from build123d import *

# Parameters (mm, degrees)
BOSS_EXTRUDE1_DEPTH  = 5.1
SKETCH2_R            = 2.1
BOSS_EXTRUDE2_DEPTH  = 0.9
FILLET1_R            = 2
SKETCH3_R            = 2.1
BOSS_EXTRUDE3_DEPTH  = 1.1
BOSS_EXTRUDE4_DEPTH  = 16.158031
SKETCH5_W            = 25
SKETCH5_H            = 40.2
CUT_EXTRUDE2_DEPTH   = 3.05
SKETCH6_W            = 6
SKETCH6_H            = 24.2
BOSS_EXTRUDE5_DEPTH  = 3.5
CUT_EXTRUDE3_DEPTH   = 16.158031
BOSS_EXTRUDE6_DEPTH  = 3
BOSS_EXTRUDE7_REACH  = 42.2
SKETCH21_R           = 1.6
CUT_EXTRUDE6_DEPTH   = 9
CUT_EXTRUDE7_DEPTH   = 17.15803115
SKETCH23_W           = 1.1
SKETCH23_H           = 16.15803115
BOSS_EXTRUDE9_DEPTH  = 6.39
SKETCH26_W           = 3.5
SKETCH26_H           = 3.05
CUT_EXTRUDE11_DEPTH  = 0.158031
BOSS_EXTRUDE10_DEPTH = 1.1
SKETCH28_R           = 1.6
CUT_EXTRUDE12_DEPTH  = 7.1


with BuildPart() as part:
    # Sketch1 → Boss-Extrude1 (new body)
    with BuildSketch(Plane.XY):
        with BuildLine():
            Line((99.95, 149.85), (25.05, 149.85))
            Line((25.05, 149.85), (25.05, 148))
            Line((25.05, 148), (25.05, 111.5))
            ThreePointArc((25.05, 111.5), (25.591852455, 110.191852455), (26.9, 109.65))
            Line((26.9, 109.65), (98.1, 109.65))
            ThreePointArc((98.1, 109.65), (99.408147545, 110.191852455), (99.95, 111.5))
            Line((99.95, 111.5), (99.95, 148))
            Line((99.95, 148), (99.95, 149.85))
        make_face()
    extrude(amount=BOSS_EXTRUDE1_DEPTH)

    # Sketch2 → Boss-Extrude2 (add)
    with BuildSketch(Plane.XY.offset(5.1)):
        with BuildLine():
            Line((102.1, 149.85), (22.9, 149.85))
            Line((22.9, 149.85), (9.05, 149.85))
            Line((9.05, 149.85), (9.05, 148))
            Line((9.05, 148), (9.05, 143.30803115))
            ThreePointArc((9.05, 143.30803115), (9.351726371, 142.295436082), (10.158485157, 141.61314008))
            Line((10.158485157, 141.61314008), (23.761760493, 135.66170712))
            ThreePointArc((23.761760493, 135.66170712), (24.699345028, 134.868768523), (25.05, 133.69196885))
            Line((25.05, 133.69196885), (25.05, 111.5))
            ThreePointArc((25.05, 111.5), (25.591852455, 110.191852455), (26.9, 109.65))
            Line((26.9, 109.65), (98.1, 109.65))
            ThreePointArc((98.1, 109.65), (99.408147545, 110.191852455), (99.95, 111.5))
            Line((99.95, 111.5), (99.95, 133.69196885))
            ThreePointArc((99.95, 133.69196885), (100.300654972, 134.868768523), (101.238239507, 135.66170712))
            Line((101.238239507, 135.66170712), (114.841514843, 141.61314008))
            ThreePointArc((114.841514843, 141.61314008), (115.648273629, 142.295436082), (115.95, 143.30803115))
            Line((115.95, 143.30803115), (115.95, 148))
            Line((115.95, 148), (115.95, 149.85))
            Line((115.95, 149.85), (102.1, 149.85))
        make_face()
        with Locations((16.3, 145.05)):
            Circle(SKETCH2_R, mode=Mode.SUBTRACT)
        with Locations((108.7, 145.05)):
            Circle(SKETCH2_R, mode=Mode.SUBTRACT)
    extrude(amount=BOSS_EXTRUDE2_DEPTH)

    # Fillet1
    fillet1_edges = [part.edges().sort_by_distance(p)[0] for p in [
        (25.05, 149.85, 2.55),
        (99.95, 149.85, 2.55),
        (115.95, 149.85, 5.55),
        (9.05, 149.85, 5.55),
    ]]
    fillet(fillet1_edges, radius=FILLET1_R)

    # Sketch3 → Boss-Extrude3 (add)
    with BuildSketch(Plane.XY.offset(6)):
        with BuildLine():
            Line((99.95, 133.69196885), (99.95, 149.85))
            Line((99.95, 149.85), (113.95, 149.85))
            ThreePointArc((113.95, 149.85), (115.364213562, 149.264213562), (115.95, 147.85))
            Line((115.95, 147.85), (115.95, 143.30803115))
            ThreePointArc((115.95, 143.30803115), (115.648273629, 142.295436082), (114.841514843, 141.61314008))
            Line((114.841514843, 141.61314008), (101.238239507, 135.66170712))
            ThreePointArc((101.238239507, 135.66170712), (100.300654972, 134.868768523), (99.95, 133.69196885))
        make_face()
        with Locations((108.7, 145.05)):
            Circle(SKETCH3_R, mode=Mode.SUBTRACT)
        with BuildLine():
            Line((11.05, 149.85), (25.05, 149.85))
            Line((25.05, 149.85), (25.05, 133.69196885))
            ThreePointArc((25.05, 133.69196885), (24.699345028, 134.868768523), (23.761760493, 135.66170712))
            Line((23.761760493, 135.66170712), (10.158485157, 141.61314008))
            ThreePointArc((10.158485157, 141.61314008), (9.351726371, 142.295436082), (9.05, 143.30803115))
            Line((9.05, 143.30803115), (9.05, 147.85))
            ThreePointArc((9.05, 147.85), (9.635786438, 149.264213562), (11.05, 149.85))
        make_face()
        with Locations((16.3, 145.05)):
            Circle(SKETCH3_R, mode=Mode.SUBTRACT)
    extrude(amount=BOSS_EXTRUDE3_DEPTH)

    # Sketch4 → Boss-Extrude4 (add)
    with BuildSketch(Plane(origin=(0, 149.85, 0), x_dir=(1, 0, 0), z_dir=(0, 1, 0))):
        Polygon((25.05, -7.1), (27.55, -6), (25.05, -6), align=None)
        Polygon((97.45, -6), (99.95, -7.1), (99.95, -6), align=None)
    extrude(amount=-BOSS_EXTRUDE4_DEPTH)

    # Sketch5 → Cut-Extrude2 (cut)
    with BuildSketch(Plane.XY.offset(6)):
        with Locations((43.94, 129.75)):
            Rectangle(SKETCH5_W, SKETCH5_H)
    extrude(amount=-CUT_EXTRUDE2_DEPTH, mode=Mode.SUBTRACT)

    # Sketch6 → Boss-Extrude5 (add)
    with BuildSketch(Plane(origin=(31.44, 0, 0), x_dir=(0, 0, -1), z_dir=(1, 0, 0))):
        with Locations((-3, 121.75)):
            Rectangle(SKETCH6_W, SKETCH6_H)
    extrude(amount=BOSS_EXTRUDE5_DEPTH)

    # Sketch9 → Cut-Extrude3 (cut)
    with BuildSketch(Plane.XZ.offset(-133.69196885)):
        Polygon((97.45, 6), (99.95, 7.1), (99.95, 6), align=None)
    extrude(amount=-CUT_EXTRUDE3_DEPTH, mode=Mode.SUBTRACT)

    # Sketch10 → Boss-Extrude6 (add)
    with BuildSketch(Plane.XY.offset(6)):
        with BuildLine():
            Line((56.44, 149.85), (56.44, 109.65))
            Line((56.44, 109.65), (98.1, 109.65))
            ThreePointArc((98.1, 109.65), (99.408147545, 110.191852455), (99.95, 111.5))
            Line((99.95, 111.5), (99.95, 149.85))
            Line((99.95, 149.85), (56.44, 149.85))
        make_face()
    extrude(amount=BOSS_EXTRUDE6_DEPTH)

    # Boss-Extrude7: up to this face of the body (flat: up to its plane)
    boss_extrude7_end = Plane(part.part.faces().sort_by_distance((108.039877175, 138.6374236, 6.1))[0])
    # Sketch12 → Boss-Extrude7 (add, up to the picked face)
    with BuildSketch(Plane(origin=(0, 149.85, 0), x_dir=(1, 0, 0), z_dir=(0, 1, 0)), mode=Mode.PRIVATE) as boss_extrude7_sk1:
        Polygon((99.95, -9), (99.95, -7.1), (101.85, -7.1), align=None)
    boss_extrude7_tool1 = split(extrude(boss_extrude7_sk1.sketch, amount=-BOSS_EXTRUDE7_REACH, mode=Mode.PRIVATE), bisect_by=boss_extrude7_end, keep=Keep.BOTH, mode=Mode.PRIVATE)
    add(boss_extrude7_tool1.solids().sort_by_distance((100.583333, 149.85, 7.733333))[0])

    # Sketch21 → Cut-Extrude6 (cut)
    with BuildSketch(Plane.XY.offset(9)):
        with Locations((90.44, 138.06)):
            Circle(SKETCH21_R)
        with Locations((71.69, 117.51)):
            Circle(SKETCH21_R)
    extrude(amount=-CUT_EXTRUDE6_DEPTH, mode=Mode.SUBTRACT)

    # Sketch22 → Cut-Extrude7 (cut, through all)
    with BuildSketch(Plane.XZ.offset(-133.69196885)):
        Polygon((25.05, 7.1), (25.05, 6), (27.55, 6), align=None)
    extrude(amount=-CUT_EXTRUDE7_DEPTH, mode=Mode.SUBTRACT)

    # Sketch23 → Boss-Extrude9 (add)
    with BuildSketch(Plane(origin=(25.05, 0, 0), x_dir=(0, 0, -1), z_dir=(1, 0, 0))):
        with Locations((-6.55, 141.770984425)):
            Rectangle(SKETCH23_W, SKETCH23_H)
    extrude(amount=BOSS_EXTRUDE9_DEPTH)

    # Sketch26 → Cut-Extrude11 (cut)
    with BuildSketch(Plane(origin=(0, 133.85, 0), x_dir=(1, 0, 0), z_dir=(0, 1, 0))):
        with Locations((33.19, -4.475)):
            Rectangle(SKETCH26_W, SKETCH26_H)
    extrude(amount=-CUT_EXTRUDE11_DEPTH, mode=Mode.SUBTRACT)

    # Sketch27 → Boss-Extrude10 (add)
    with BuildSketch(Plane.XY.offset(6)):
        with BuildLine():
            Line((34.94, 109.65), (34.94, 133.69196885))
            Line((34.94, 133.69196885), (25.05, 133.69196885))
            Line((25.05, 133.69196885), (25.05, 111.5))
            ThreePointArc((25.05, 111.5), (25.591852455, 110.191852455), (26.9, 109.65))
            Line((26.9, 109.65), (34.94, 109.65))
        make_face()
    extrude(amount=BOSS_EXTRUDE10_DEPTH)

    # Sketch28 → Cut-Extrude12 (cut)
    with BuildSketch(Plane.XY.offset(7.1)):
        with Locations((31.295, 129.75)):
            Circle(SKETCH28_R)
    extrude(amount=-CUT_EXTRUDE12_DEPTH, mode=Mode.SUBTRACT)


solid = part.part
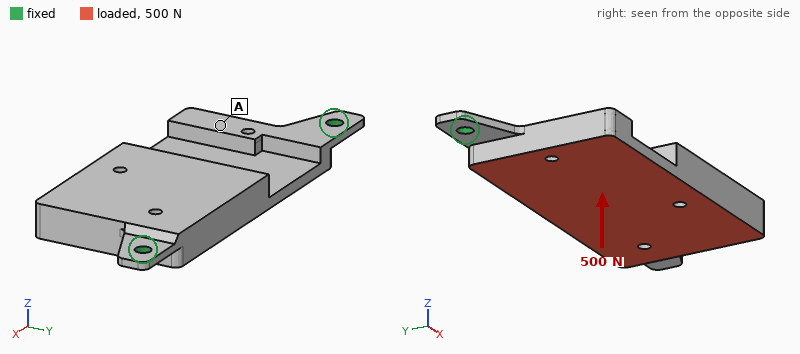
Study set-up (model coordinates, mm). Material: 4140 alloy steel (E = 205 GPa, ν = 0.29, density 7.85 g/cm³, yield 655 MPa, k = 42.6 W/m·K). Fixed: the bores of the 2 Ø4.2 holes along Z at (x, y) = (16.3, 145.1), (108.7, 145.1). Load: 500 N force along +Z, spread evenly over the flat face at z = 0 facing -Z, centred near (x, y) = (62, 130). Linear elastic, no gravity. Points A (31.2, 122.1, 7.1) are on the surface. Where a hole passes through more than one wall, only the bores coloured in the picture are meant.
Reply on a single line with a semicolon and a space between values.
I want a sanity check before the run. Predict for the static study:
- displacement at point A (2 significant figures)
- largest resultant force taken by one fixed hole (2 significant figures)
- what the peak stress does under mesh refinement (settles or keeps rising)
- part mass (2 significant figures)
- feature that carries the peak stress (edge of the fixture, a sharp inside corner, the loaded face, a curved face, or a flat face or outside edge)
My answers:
0.19 mm; 740 N; keeps rising; 170 g; edge of the fixture
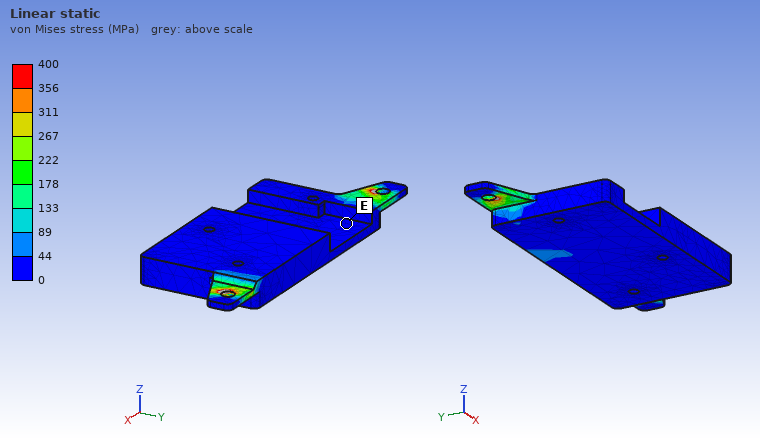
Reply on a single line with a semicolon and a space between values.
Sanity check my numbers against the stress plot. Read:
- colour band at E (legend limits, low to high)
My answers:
0 to 44 MPa
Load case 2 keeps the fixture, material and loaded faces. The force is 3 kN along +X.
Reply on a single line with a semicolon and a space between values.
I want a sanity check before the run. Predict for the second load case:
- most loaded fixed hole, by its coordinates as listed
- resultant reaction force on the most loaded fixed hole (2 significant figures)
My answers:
(108.7, 145.1); 2.1 kN
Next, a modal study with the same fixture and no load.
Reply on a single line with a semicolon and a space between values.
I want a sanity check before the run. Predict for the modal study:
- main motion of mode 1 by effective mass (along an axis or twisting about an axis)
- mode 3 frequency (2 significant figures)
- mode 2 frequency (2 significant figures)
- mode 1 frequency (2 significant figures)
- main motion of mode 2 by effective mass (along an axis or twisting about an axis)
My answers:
along Z; 3200 Hz; 2400 Hz; 610 Hz; along Z
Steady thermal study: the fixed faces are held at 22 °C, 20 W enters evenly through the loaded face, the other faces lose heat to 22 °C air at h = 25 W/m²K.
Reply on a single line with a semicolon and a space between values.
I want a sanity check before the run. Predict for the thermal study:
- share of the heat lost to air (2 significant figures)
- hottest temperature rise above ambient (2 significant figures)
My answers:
43 %; 70 K
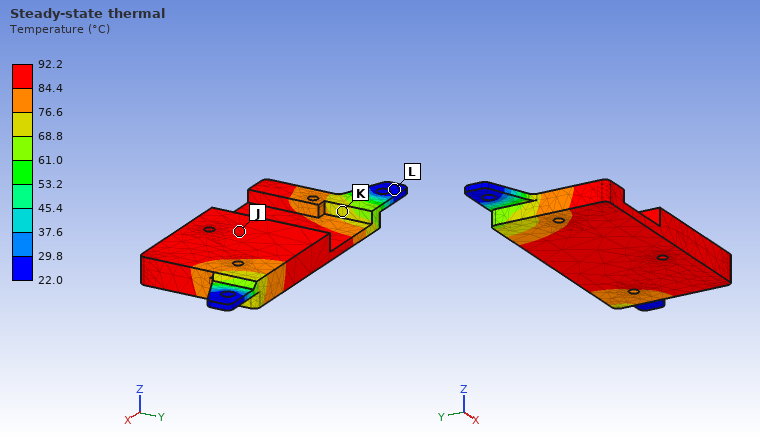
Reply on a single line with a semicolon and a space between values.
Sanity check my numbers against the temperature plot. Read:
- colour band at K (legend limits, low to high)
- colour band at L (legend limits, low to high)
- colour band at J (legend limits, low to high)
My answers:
68.8 to 76.6 °C; 22.0 to 29.8 °C; 84.4 to 92.2 °C
